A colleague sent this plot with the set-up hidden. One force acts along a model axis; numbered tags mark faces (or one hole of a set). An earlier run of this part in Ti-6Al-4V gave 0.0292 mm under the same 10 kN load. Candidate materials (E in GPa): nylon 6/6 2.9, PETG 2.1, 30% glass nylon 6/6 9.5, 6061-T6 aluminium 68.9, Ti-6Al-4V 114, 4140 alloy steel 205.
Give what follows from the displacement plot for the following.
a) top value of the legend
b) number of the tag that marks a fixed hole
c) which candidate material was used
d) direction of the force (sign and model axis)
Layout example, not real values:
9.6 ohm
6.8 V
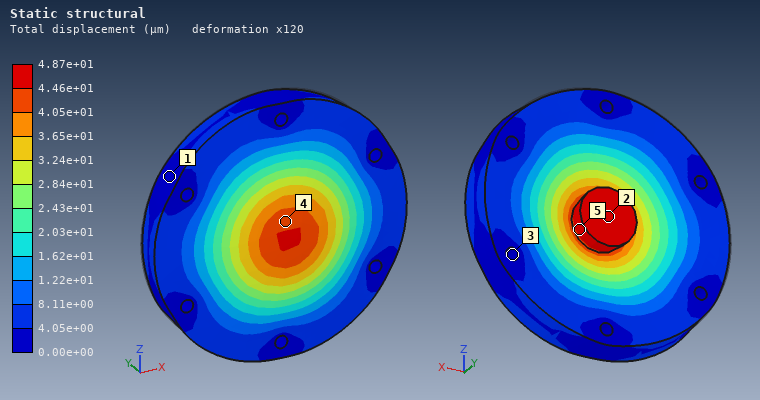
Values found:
4.87e+01 µm
3
6061-T6 aluminium
-Y
